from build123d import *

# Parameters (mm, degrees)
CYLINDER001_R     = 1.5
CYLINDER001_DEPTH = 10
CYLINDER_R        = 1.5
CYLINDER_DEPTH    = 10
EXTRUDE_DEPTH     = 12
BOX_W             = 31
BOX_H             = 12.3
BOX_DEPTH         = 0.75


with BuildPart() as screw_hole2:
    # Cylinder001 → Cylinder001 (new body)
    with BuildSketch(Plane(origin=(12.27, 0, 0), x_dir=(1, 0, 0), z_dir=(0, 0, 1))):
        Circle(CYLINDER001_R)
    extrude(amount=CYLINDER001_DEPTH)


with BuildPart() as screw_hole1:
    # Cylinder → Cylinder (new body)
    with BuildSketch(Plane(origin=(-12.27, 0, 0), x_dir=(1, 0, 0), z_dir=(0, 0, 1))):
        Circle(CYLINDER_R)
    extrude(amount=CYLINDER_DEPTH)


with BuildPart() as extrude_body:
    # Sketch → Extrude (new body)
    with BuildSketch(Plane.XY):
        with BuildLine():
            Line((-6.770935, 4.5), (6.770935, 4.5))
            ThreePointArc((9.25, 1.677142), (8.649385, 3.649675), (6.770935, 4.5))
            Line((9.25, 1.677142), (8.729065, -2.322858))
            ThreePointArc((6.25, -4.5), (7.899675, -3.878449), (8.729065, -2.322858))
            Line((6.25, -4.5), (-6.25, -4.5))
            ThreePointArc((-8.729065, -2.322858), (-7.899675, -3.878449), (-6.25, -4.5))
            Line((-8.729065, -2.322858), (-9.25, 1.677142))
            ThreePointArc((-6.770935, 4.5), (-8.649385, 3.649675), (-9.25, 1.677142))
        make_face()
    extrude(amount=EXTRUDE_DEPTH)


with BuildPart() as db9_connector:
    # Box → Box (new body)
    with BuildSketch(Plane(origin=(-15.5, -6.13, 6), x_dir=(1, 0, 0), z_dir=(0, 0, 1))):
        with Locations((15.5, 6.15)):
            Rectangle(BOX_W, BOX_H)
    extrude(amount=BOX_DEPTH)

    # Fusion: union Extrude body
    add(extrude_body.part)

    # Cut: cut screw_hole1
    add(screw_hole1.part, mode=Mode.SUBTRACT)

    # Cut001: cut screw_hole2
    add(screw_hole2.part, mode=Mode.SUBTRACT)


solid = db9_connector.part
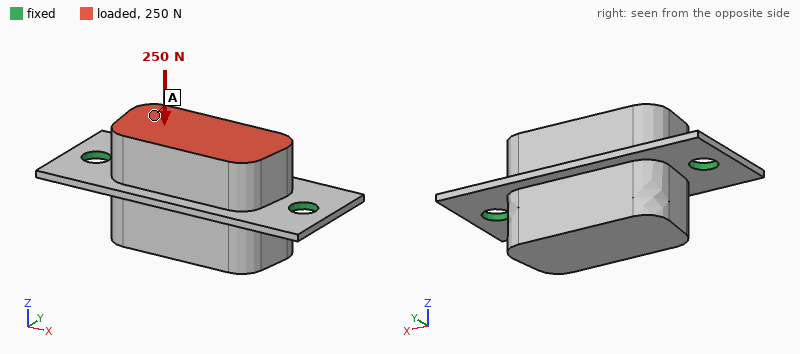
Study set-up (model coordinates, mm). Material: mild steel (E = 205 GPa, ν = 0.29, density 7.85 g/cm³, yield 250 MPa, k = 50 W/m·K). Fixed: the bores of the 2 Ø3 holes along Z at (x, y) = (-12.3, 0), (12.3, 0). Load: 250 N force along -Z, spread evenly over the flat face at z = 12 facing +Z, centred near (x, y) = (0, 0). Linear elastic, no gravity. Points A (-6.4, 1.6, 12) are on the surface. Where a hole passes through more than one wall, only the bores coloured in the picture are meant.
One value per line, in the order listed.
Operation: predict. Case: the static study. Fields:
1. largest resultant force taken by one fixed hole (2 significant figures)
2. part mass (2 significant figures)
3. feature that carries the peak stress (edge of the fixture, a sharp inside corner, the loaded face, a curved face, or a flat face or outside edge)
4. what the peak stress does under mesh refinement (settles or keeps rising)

130 N
16 g
edge of the fixture
keeps rising
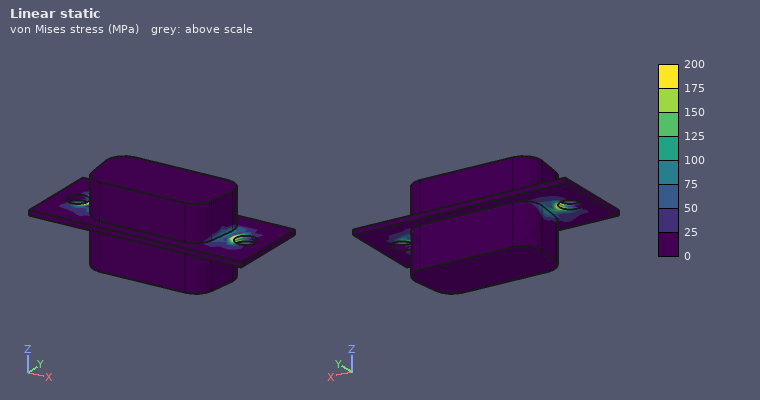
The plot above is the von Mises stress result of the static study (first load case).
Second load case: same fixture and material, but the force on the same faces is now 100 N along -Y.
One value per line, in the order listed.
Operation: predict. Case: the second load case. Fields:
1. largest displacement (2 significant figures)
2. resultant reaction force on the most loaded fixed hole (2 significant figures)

21 µm
50 N
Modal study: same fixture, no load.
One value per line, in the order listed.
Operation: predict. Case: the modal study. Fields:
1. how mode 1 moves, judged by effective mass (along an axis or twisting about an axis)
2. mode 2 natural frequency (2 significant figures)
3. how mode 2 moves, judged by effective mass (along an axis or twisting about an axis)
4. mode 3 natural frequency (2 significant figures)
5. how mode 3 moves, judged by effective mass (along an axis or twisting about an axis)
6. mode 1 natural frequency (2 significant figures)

twisting about X
11 kHz
along Z
17 kHz
twisting about Y
4300 Hz
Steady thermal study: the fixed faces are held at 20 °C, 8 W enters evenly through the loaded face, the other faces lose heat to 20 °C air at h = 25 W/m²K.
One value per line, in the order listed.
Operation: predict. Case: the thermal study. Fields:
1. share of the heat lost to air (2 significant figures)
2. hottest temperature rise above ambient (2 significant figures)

11 %
40 K
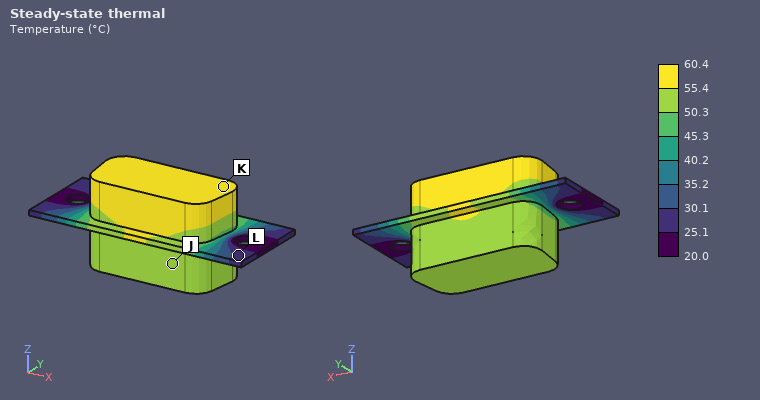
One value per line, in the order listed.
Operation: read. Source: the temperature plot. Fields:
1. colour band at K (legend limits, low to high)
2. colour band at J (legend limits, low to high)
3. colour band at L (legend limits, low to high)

55.4 to 60.4 °C
50.3 to 55.4 °C
25.1 to 30.1 °C
